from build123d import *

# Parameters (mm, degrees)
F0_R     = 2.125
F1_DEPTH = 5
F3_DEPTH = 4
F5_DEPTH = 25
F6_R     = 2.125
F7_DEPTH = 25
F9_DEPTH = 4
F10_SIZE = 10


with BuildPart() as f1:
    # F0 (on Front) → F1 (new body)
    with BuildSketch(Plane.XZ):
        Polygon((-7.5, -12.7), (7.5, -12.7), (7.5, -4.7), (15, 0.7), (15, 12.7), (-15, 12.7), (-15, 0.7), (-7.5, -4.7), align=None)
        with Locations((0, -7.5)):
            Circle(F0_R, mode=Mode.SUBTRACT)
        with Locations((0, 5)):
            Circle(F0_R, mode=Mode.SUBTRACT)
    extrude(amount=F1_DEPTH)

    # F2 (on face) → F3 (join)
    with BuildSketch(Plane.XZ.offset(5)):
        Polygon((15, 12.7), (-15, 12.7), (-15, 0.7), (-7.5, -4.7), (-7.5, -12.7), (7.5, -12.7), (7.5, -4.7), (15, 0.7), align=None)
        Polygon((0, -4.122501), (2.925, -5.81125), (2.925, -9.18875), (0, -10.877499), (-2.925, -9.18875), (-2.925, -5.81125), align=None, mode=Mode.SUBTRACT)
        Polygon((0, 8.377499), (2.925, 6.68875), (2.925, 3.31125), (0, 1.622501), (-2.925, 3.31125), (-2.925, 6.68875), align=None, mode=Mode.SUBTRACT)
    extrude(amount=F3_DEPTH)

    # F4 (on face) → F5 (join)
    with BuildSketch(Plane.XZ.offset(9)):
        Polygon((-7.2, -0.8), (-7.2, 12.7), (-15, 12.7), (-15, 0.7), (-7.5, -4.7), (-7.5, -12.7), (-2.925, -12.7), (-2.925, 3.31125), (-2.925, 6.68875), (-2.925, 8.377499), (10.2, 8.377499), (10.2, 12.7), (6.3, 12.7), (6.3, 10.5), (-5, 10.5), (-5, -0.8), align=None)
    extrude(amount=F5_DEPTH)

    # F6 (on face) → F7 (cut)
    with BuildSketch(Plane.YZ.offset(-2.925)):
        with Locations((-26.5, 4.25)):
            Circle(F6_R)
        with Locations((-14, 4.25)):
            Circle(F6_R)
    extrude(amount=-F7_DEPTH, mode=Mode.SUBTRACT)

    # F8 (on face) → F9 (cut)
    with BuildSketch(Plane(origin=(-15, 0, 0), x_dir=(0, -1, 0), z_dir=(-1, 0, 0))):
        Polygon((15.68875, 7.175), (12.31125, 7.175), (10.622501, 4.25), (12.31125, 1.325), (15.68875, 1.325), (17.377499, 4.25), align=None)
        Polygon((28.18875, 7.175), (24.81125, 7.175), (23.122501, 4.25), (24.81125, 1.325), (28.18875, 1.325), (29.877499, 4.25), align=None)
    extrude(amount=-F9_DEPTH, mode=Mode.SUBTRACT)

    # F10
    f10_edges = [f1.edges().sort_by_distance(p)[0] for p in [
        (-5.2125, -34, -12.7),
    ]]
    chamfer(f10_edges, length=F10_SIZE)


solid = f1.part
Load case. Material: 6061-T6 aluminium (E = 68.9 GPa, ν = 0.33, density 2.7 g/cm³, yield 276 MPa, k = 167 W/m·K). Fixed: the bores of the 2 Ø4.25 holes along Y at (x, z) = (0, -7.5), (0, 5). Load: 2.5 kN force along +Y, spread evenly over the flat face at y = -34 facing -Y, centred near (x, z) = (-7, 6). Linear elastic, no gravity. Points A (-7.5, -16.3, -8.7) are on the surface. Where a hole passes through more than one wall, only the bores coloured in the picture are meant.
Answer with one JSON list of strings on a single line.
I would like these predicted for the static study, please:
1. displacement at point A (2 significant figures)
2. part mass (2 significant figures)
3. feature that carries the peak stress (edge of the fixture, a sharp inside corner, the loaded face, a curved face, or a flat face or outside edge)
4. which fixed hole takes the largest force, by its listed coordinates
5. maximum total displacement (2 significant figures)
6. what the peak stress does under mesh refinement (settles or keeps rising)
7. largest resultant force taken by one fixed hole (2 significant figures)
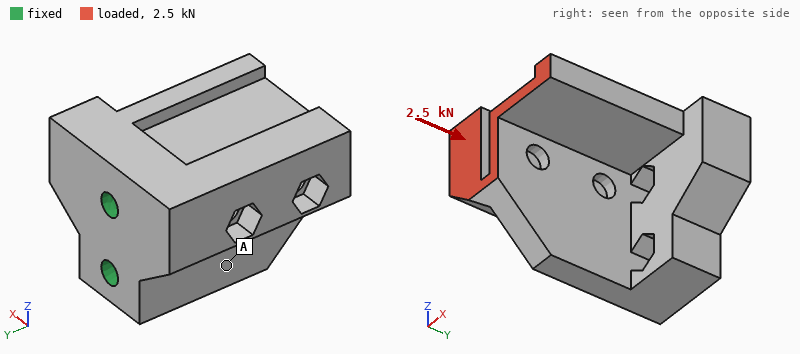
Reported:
["25 µm", "27 g", "edge of the fixture", "(0, 5)", "84 µm", "keeps rising", "2.3 kN"]
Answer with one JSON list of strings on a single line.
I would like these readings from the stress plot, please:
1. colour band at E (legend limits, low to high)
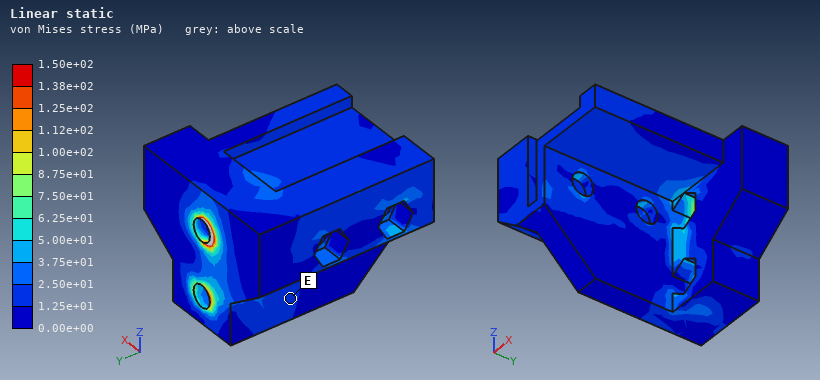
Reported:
["1.25e+01 to 2.50e+01 MPa"]
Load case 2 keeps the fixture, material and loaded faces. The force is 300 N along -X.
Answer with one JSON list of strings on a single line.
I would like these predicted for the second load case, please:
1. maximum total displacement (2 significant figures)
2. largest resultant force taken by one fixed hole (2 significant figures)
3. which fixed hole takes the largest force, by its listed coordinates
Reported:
["69 µm", "260 N", "(0, 5)"]
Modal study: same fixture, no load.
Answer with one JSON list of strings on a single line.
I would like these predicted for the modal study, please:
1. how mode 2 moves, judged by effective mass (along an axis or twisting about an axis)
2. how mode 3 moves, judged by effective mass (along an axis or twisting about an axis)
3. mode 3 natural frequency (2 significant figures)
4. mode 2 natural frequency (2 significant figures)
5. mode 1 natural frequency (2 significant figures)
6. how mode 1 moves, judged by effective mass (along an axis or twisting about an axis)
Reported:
["along Z", "along Z", "11 kHz", "7200 Hz", "5100 Hz", "along X"]
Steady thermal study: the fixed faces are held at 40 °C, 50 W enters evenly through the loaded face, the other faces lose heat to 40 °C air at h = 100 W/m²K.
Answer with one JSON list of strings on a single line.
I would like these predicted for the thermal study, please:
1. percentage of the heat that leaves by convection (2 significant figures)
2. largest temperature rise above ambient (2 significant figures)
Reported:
["19 %", "51 K"]
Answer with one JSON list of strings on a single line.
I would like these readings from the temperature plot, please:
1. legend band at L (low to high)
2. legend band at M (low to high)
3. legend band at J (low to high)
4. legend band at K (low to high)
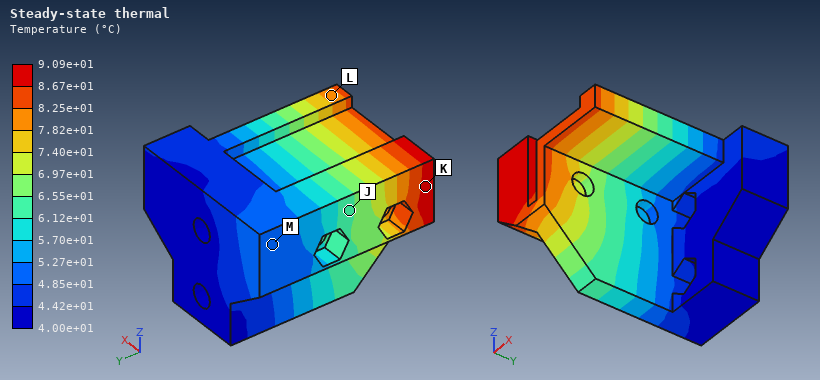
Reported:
["7.82e+01 to 8.25e+01 °C", "4.85e+01 to 5.27e+01 °C", "6.12e+01 to 6.55e+01 °C", "8.67e+01 to 9.09e+01 °C"]
